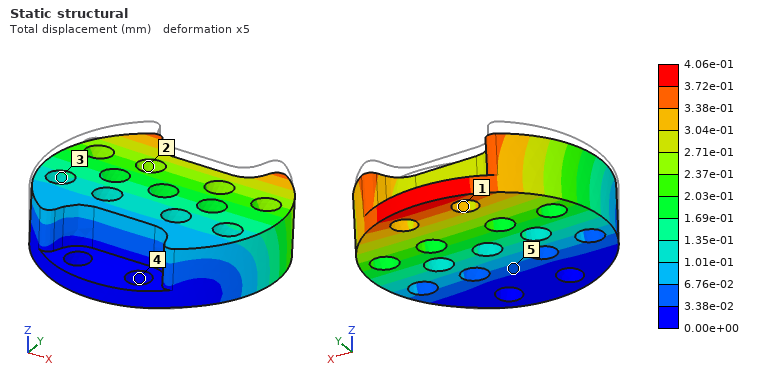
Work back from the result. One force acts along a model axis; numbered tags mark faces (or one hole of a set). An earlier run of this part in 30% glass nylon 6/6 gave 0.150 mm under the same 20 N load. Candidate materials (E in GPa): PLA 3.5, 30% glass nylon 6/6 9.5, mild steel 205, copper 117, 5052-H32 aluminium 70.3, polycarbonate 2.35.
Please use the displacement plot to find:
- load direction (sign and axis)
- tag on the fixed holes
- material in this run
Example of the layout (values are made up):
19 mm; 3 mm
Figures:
-Z; 4; PLA
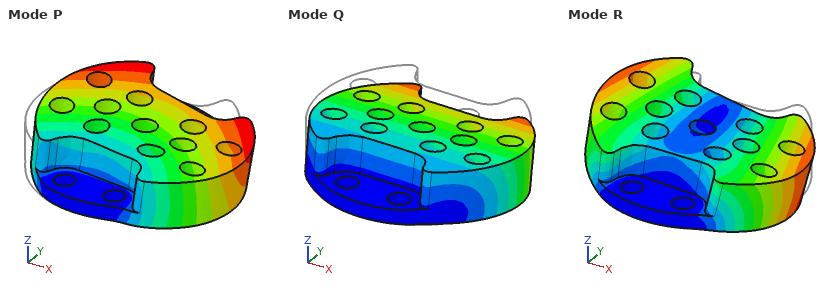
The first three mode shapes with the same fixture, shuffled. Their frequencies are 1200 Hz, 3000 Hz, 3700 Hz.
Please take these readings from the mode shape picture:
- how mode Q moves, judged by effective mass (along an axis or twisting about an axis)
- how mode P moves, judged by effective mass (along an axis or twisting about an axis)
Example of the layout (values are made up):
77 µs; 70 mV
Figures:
along Z; along X
